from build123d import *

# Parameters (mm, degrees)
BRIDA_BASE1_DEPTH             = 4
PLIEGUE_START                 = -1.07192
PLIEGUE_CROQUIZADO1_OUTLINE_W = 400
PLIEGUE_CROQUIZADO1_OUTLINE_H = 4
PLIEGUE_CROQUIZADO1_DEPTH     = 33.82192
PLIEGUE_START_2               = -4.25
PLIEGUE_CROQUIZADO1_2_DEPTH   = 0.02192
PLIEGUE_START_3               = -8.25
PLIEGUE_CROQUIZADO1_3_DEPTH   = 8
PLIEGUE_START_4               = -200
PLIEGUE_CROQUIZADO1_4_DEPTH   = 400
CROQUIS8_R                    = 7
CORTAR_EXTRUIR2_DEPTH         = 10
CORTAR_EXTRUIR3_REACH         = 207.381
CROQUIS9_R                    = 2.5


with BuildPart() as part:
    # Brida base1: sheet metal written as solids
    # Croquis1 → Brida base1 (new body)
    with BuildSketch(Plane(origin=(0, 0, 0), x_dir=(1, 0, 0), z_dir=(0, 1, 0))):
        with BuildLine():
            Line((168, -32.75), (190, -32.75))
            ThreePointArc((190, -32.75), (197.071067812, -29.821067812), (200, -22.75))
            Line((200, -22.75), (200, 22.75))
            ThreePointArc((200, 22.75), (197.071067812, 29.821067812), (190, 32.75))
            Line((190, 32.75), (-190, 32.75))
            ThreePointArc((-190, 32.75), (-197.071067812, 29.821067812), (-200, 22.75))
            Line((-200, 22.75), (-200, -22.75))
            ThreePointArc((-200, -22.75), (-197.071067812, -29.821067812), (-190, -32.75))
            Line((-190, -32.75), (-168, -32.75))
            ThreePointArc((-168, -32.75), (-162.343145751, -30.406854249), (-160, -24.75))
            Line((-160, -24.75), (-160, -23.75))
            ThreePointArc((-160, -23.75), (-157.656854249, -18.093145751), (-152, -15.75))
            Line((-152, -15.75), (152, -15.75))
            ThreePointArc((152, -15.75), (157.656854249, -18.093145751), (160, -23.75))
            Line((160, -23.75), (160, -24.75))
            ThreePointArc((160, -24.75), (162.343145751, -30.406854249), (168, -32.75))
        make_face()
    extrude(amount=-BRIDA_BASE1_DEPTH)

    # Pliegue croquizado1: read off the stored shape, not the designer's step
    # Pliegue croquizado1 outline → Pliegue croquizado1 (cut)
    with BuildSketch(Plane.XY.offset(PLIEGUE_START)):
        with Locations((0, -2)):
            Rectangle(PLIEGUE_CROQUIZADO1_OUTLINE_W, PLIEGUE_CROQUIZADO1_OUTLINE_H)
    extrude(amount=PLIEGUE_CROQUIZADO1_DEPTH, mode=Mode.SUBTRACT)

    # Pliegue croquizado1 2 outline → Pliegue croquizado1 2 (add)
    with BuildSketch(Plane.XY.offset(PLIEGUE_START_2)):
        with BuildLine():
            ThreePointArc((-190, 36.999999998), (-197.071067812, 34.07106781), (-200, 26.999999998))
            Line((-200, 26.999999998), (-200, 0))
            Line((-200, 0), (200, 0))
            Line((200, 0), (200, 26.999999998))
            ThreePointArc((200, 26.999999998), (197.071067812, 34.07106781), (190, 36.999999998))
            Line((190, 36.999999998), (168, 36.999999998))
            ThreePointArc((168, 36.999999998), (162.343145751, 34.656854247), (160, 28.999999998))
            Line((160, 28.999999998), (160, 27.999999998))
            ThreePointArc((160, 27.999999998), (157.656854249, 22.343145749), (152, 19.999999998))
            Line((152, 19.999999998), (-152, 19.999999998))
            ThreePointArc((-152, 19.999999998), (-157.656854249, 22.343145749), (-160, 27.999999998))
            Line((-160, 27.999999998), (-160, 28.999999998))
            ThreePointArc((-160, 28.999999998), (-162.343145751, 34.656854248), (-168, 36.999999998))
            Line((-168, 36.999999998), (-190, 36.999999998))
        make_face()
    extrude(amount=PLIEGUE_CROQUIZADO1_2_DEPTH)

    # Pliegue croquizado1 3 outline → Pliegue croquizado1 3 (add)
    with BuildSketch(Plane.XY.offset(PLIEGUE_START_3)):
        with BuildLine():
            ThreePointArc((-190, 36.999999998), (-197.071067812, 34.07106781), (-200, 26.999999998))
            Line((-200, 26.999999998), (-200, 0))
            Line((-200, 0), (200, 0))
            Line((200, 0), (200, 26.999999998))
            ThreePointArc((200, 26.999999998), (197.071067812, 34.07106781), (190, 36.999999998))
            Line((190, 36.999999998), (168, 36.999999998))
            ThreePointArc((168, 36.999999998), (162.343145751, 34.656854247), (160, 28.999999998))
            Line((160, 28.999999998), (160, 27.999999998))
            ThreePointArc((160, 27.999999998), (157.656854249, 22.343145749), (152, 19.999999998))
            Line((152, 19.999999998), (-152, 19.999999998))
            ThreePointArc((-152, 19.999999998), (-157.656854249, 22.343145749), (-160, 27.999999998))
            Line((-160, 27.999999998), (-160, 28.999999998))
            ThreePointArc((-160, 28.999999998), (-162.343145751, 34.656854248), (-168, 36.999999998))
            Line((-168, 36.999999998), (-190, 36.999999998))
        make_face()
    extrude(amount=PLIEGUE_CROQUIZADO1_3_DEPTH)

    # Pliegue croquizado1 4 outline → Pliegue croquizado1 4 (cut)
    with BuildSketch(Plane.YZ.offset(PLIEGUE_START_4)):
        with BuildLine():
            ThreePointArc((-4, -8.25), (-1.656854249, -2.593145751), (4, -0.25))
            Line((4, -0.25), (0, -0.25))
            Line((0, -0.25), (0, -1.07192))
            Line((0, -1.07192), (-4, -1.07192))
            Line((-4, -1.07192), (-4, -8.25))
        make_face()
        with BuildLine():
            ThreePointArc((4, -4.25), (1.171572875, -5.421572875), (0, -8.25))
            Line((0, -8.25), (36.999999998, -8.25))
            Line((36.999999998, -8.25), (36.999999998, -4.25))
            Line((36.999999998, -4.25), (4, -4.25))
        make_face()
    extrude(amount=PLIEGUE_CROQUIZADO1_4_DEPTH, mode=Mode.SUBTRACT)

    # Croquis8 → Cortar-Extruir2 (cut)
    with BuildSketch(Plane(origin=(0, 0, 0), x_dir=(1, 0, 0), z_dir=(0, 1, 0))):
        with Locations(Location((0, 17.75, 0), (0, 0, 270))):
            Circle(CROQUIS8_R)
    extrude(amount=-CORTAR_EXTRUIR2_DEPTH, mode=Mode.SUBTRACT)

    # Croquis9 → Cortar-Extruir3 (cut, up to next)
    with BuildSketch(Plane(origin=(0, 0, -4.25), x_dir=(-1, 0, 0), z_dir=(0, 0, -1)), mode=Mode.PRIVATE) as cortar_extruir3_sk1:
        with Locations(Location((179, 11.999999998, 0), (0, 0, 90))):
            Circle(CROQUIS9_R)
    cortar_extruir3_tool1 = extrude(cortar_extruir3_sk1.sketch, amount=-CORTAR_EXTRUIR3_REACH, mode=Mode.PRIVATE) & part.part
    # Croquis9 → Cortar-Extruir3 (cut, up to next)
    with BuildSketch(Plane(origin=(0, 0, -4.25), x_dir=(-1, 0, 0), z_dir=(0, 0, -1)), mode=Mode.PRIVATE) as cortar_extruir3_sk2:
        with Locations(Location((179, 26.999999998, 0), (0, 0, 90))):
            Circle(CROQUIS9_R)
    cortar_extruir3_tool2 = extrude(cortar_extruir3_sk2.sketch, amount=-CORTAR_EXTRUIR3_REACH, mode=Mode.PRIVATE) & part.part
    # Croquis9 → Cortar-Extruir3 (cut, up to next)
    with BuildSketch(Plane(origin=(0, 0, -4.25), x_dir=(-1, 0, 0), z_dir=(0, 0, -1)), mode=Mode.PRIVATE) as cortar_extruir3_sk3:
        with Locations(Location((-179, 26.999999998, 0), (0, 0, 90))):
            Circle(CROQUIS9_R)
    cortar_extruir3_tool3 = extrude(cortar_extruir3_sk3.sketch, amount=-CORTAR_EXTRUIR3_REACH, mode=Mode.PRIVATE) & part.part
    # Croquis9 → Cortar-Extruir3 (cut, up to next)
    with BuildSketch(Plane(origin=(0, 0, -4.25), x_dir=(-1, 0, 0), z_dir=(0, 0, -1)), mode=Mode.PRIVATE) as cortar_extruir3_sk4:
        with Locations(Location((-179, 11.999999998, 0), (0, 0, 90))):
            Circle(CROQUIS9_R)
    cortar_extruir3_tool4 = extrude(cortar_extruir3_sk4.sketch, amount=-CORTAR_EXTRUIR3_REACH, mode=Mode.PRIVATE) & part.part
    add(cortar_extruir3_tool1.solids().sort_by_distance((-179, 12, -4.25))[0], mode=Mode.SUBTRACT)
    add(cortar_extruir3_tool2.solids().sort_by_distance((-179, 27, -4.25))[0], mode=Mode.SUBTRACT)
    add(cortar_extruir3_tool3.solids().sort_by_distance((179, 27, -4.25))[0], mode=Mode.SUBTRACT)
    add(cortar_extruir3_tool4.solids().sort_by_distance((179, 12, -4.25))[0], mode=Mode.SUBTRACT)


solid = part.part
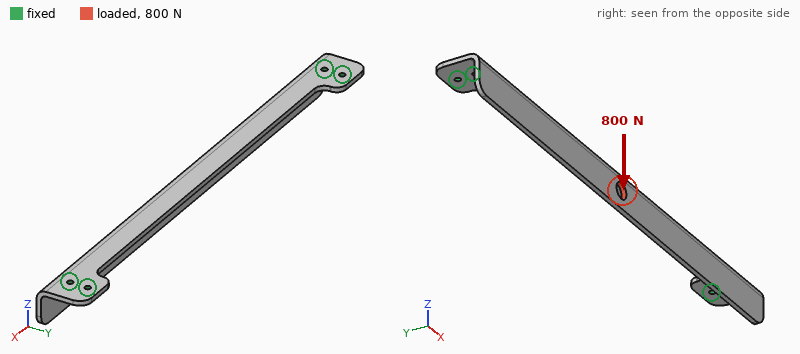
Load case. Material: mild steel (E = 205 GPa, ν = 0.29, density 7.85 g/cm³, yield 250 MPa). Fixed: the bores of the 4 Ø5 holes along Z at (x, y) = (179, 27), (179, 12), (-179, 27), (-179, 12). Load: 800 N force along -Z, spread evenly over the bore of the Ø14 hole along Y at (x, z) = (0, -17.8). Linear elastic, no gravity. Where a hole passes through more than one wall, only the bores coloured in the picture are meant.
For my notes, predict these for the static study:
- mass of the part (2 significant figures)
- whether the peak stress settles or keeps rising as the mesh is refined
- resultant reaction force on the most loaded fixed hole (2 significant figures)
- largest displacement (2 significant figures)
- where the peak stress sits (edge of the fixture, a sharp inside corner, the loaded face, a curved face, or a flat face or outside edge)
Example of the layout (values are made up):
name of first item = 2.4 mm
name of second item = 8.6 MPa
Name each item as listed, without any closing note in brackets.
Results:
mass of the part = 660 g
whether the peak stress settles or keeps rising as the mesh is refined = keeps rising
resultant reaction force on the most loaded fixed hole = 2.2 kN
largest displacement = 0.21 mm
where the peak stress sits = edge of the fixture
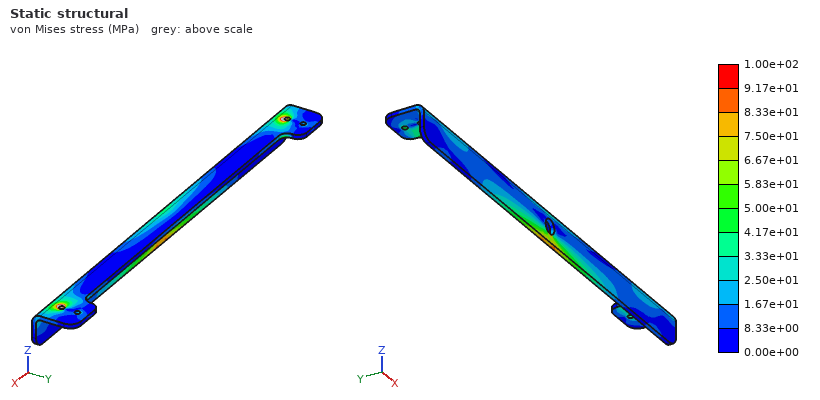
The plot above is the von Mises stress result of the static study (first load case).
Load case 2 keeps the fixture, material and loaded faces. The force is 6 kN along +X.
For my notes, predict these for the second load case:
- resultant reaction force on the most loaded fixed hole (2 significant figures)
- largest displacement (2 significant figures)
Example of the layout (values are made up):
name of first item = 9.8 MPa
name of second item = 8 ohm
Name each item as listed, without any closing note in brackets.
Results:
resultant reaction force on the most loaded fixed hole = 3.2 kN
largest displacement = 20 µm
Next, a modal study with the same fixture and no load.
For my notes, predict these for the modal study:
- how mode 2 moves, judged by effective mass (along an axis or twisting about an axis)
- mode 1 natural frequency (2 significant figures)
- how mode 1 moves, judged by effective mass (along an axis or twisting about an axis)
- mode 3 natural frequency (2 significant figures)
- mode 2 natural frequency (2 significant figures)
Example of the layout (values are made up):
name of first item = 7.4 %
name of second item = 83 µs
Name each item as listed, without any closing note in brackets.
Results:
how mode 2 moves, judged by effective mass = along Z
mode 1 natural frequency = 550 Hz
how mode 1 moves, judged by effective mass = along Y
mode 3 natural frequency = 1200 Hz
mode 2 natural frequency = 670 Hz
